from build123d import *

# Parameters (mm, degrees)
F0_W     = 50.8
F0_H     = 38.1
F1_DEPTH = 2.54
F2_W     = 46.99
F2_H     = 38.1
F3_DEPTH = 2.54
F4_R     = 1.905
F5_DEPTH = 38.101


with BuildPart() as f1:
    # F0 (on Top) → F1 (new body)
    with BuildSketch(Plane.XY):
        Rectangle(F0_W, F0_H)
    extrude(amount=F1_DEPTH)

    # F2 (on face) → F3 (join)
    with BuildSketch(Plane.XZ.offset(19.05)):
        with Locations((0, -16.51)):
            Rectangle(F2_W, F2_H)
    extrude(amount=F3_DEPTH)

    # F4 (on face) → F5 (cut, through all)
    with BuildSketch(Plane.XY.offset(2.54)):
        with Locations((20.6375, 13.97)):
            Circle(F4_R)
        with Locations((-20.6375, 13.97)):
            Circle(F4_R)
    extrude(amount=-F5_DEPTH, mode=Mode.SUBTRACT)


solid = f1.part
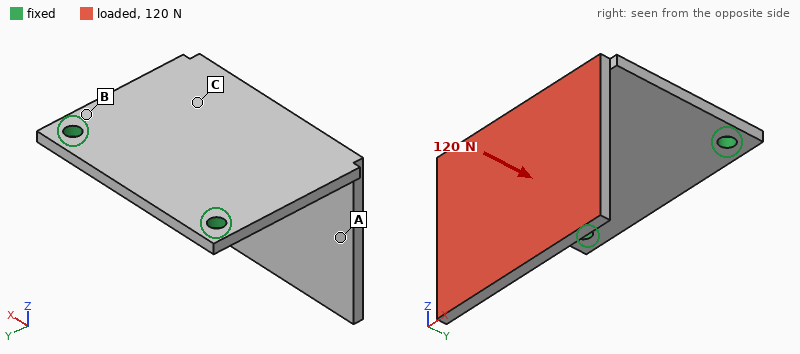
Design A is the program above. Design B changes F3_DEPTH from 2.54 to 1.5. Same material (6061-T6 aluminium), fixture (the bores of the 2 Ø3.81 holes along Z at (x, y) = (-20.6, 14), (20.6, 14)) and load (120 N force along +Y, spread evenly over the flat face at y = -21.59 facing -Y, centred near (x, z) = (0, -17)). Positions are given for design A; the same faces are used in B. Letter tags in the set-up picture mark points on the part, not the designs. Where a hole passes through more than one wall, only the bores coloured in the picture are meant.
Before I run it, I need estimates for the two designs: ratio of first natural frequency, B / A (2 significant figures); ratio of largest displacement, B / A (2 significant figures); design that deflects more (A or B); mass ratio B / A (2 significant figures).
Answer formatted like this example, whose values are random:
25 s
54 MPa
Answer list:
1.2
1.6
B
0.80
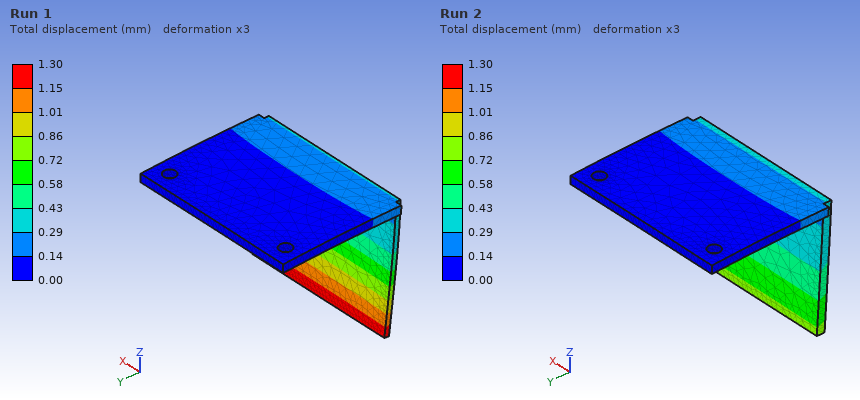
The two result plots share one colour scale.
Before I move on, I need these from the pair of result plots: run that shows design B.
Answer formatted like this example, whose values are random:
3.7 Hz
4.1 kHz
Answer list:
Run 1
